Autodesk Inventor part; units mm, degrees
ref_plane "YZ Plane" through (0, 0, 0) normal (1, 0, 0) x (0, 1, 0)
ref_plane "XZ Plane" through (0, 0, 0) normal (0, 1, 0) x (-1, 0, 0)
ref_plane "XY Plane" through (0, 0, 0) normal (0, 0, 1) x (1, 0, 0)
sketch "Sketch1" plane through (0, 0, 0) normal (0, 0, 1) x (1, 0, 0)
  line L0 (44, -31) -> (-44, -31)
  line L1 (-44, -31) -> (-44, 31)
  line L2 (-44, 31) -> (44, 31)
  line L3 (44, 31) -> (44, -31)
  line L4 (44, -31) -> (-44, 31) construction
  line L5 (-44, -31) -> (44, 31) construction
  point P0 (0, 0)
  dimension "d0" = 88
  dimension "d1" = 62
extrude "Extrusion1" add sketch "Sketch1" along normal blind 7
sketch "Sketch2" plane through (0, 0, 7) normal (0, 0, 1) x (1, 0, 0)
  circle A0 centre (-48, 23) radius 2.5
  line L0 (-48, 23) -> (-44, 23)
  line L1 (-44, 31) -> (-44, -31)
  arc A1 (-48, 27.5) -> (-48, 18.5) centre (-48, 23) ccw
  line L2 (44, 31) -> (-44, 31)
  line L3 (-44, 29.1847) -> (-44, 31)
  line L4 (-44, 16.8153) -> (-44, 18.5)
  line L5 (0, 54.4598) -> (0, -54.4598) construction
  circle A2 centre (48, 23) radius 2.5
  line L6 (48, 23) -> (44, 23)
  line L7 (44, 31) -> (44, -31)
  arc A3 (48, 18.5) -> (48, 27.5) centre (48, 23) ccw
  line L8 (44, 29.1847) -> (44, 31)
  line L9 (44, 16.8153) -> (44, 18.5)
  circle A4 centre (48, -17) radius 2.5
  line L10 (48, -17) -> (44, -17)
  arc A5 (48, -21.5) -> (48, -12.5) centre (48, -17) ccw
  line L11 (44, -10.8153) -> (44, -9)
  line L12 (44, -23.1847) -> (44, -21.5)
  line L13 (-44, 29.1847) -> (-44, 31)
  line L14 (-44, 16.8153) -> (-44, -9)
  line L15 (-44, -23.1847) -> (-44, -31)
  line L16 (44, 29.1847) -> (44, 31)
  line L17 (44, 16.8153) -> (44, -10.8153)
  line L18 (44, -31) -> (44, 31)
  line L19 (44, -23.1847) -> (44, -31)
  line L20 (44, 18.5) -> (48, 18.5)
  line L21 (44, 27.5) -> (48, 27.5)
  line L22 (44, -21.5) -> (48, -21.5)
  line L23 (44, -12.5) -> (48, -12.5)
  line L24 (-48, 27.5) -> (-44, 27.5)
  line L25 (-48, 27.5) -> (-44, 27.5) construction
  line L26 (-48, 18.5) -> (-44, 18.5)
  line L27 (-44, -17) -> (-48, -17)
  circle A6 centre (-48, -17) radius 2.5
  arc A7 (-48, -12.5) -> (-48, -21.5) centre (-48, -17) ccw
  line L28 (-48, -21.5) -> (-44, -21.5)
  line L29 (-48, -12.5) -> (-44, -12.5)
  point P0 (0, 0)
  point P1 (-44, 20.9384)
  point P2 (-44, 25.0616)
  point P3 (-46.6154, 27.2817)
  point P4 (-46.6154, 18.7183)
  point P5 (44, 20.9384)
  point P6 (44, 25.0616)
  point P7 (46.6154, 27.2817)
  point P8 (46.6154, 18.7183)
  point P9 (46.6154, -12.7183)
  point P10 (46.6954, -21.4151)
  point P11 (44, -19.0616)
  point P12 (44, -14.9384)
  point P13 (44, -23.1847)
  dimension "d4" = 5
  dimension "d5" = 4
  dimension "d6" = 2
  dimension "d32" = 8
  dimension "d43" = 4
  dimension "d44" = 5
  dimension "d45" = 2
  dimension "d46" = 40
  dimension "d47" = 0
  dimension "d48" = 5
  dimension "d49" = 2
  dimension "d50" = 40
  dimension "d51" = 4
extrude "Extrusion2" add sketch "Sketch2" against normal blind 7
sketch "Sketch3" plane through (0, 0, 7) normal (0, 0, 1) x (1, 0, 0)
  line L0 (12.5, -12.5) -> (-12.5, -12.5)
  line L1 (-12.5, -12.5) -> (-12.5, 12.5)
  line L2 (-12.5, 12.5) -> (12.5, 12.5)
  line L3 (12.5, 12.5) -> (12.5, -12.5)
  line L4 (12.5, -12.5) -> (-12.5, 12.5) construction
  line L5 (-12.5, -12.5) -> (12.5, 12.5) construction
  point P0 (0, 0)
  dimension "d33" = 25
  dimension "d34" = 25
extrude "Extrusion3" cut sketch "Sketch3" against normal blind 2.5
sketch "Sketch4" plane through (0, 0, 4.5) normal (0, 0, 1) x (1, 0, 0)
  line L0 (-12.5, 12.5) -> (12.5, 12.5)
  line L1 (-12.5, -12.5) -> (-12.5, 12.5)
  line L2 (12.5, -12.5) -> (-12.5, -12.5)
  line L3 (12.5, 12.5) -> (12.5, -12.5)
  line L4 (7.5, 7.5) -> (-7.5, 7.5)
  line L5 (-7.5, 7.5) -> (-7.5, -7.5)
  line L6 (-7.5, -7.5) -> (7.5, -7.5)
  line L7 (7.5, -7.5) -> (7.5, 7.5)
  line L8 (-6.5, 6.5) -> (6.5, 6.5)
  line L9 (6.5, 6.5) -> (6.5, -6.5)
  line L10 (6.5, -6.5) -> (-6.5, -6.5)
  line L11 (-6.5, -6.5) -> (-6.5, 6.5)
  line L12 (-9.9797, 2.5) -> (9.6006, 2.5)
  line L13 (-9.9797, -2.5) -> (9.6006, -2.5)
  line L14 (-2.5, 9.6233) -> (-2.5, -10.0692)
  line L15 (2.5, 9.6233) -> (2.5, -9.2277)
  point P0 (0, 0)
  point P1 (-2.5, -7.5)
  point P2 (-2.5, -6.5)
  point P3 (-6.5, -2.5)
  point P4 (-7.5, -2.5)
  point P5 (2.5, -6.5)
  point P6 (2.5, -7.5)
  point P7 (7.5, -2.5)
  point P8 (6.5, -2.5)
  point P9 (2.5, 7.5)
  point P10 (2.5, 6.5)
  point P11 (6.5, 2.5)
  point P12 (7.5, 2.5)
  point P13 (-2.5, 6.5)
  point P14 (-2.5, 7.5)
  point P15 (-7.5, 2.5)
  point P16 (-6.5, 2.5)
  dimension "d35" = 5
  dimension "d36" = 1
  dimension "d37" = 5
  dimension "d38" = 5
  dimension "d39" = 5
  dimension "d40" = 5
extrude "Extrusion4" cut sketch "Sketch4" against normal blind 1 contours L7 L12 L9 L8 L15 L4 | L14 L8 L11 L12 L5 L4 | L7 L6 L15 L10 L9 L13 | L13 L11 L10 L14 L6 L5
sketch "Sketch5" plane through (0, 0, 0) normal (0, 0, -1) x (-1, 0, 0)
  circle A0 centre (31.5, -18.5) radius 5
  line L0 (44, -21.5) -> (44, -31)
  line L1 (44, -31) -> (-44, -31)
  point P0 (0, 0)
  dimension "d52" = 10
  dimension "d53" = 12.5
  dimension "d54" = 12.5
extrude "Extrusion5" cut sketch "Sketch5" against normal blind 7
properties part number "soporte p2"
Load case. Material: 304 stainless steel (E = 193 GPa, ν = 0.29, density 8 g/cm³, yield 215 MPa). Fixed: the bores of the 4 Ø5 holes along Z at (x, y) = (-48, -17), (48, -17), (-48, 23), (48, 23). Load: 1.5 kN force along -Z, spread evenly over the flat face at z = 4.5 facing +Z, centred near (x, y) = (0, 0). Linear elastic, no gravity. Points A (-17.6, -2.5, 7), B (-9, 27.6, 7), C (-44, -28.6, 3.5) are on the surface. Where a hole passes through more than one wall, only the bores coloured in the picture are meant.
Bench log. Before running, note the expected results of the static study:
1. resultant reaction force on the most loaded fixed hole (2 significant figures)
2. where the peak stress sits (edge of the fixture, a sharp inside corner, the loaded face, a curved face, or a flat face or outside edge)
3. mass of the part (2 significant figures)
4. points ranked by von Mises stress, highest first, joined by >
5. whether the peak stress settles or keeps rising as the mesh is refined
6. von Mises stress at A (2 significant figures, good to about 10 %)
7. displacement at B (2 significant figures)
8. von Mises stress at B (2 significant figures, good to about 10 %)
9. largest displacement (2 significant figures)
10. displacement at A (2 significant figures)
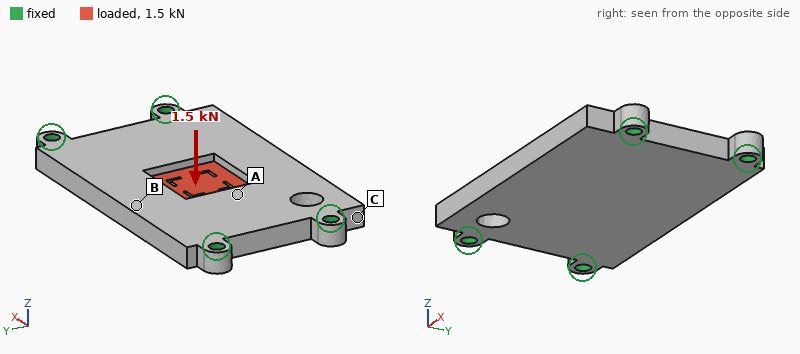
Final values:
490 N
edge of the fixture
300 g
B > A > C
keeps rising
16 MPa
26 µm
32 MPa
38 µm
27 µm
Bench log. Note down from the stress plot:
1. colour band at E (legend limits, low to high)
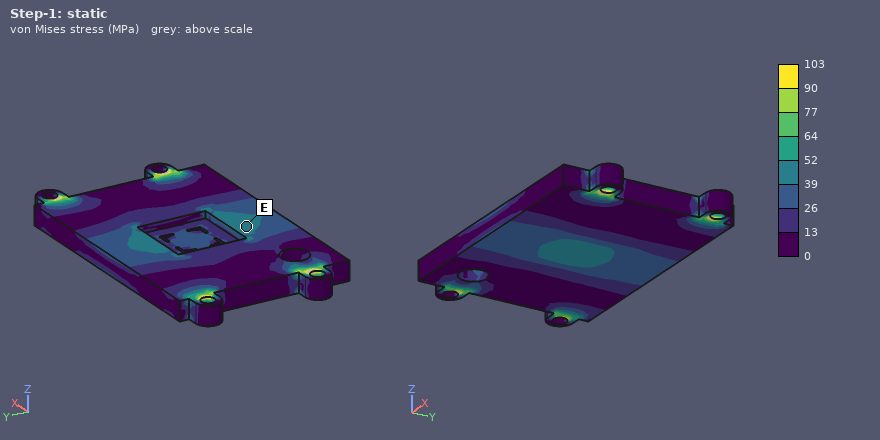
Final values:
39 to 52 MPa
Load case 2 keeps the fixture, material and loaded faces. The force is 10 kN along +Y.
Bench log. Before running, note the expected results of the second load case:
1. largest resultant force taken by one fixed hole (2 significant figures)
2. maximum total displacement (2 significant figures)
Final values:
3.2 kN
17 µm
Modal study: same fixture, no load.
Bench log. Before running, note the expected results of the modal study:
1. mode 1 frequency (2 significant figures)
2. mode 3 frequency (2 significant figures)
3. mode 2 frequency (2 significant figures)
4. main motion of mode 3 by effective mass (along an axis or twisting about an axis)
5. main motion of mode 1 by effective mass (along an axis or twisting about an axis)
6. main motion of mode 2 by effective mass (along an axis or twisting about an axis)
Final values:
3000 Hz
8300 Hz
4600 Hz
twisting about Y
along Z
twisting about X
